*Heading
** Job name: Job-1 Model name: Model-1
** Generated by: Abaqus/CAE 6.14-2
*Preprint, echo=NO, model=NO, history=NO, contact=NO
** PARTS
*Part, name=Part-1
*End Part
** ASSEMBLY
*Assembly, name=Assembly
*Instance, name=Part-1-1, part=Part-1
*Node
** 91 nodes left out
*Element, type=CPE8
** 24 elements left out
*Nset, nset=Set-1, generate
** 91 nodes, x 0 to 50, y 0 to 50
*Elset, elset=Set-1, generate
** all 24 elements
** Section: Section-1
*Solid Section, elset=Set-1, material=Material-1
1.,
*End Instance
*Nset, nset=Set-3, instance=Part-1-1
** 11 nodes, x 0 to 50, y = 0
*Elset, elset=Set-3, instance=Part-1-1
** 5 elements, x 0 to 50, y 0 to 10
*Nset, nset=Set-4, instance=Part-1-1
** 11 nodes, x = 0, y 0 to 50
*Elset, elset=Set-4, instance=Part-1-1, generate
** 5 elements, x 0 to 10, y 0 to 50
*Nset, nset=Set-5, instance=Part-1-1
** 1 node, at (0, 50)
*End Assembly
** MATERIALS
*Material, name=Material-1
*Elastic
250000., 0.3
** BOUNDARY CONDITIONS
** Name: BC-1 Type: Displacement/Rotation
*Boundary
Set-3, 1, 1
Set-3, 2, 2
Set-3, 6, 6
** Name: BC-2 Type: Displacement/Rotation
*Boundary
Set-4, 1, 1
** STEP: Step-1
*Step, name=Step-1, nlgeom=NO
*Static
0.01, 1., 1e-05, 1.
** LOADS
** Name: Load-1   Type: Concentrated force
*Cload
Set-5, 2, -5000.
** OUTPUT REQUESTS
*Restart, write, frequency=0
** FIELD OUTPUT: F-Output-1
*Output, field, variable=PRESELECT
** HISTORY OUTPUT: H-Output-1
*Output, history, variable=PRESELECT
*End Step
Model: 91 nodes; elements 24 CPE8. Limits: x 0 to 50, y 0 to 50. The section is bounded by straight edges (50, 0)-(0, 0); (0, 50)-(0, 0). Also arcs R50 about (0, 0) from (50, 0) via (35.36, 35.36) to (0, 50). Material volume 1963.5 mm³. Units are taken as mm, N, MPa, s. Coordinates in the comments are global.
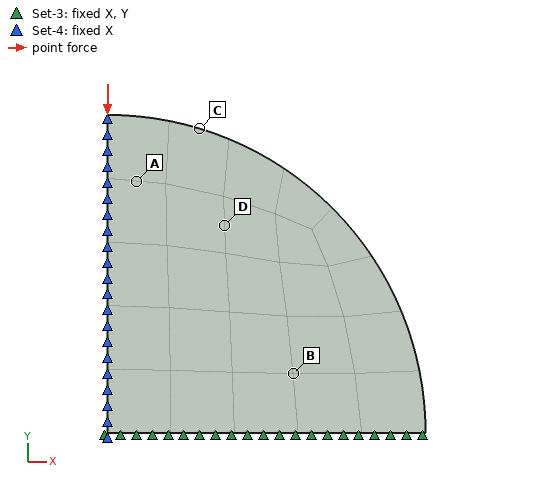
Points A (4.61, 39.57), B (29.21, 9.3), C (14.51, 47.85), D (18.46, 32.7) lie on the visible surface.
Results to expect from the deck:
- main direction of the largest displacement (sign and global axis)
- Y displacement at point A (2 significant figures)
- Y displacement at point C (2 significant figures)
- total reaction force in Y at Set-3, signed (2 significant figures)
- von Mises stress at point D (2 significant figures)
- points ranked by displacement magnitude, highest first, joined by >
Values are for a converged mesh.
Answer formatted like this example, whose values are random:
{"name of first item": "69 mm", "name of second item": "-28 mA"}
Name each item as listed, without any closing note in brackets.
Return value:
{"main direction of the largest displacement": "-Y", "Y displacement at point A": "-0.037 mm", "Y displacement at point C": "-0.019 mm", "total reaction force in Y at Set-3, signed": "5000 N", "von Mises stress at point D": "130 MPa", "points ranked by displacement magnitude, highest first, joined by >": "A > C > D > B"}
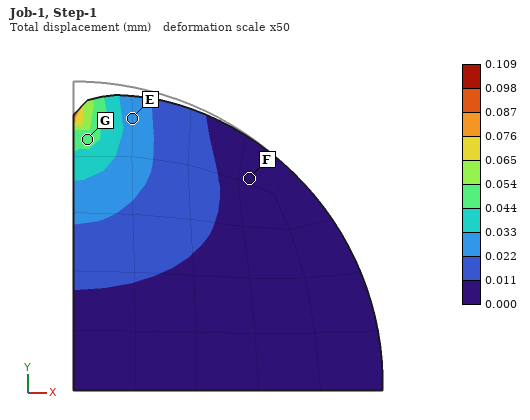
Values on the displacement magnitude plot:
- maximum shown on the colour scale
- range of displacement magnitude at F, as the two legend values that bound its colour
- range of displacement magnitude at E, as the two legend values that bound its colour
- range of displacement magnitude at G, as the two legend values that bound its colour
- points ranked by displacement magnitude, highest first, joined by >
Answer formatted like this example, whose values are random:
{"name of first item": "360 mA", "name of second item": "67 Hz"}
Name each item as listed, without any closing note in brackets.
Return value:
{"maximum shown on the colour scale": "0.109 mm", "range of displacement magnitude at F, as the two legend values that bound its colour": "0.000 to 0.011 mm", "range of displacement magnitude at E, as the two legend values that bound its colour": "0.022 to 0.033 mm", "range of displacement magnitude at G, as the two legend values that bound its colour": "0.044 to 0.054 mm", "points ranked by displacement magnitude, highest first, joined by >": "G > E > F"}
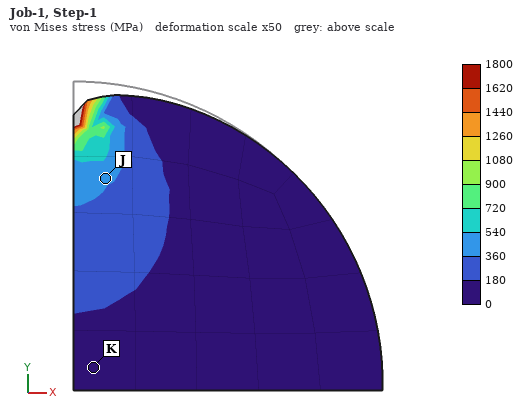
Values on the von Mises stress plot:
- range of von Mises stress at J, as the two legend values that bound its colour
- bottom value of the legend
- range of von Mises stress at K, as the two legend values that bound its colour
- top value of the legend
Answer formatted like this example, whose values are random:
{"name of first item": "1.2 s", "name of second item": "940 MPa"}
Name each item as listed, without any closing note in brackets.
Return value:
{"range of von Mises stress at J, as the two legend values that bound its colour": "360 to 540 MPa", "bottom value of the legend": "0 MPa", "range of von Mises stress at K, as the two legend values that bound its colour": "0 to 180 MPa", "top value of the legend": "1800 MPa"}
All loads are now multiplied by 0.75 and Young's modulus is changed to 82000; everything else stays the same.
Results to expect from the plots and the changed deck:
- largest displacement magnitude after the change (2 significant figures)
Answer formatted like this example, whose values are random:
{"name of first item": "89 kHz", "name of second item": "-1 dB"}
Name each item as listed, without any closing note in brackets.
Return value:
{"largest displacement magnitude after the change": "0.25 mm"}
